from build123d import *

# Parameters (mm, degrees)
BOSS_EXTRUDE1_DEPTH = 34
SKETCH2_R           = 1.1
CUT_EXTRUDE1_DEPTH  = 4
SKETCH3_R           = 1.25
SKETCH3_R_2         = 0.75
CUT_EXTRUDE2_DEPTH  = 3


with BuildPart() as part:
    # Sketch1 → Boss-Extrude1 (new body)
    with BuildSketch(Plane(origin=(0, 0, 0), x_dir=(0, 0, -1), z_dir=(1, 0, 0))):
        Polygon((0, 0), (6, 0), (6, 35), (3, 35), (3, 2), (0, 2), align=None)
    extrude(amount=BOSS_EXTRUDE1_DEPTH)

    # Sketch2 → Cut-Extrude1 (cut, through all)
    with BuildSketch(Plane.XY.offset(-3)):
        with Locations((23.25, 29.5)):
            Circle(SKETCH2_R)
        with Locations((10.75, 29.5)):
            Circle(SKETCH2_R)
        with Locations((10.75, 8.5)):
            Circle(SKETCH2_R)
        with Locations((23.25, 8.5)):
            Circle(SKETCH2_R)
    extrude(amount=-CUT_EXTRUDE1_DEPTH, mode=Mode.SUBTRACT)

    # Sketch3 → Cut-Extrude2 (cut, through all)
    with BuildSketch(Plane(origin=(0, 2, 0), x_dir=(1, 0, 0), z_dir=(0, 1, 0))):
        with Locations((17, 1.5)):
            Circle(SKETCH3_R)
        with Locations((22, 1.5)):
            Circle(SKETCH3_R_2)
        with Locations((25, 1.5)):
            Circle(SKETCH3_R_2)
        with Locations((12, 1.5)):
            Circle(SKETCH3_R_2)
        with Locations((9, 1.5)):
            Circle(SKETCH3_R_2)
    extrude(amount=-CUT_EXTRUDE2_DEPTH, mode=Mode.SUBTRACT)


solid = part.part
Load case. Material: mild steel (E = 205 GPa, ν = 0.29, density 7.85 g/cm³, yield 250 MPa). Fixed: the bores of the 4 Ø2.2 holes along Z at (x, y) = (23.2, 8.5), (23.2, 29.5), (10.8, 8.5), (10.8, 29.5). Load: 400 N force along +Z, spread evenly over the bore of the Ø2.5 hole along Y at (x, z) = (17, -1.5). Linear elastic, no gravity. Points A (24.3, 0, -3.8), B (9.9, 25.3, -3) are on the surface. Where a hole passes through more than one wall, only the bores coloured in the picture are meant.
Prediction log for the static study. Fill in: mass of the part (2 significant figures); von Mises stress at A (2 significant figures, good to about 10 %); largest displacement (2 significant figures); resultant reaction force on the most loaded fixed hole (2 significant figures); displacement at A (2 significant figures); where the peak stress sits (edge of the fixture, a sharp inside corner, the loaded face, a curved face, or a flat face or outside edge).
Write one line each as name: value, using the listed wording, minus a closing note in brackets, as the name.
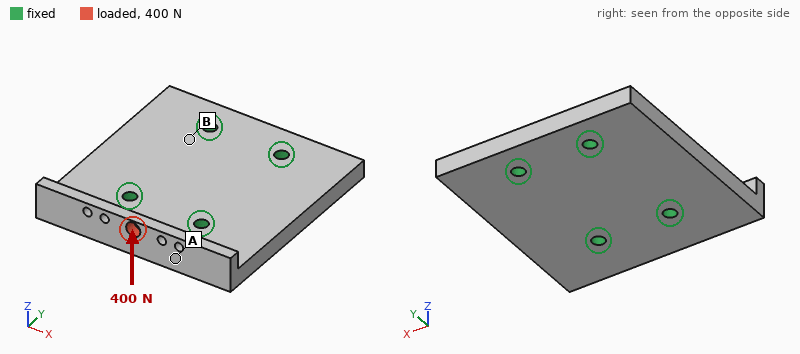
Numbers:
mass of the part: 29 g
von Mises stress at A: 28 MPa
largest displacement: 12 µm
resultant reaction force on the most loaded fixed hole: 220 N
displacement at A: 6.1 µm
where the peak stress sits: a flat face or outside edge
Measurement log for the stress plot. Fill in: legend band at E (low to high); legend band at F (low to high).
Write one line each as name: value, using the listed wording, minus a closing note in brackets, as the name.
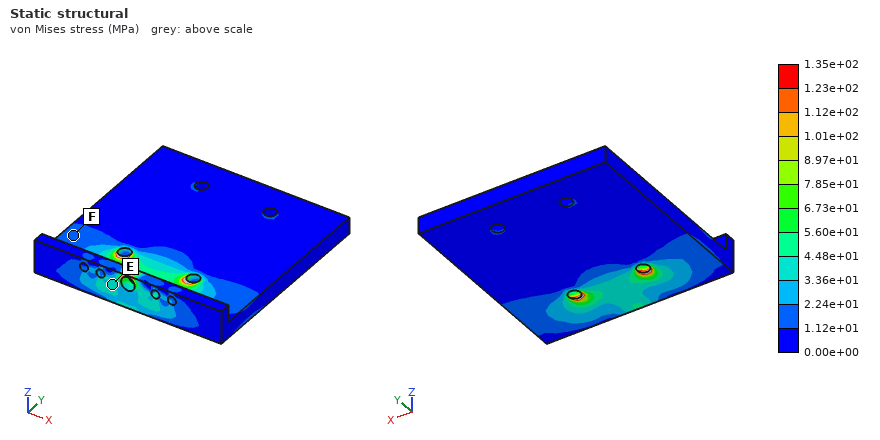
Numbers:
legend band at E: 3.36e+01 to 4.48e+01 MPa
legend band at F: 1.12e+01 to 2.24e+01 MPa
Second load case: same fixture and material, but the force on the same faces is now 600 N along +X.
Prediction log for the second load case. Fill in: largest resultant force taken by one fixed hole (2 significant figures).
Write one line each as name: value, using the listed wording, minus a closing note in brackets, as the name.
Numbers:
largest resultant force taken by one fixed hole: 390 N
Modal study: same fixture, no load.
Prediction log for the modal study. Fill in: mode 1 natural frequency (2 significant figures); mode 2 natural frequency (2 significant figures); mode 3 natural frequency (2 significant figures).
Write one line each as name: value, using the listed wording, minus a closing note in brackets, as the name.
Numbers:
mode 1 natural frequency: 17 kHz
mode 2 natural frequency: 17 kHz
mode 3 natural frequency: 18 kHz
